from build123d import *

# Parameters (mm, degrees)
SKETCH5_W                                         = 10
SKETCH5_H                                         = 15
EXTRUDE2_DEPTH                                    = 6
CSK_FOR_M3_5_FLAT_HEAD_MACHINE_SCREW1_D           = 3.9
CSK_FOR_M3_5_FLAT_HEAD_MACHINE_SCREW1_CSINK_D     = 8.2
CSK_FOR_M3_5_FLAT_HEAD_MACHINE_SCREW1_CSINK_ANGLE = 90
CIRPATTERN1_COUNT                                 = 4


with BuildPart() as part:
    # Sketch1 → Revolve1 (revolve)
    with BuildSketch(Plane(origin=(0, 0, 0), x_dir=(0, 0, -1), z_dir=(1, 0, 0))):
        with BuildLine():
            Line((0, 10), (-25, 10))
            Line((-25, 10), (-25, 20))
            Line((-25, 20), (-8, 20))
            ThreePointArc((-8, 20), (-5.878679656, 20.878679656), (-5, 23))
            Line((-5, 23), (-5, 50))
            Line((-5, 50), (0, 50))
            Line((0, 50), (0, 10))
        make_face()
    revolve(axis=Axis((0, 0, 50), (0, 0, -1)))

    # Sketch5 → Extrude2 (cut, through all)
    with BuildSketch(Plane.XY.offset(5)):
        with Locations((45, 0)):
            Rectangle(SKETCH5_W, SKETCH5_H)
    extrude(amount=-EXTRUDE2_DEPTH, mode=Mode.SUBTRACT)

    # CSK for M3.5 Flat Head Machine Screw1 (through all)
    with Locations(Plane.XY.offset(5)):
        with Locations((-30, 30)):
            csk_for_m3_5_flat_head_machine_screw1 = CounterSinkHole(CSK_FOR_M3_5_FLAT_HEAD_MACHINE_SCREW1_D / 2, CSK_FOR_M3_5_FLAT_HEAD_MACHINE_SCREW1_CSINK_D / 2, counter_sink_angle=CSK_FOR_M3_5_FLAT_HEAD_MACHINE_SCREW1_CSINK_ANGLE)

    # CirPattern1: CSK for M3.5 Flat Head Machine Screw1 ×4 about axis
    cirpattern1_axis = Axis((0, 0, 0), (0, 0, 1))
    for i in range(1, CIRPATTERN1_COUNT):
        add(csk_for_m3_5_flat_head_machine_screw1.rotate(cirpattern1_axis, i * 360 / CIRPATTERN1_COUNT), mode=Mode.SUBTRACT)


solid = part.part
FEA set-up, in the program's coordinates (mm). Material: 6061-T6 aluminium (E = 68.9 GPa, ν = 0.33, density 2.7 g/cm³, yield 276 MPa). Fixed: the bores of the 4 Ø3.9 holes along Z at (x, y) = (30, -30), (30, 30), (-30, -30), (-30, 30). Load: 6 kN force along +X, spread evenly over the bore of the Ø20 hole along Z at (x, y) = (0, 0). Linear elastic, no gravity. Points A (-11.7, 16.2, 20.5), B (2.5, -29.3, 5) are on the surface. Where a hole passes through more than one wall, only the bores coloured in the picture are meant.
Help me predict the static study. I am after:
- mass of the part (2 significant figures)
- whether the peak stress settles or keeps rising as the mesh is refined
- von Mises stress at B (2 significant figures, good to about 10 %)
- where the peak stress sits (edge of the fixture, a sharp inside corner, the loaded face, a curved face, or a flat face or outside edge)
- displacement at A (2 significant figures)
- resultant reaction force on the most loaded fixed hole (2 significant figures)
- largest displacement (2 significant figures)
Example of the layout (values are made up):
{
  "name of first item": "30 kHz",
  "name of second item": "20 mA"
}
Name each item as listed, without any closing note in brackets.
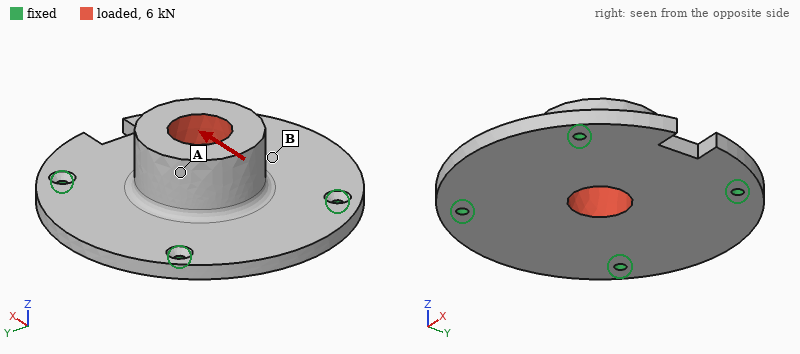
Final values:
{
  "mass of the part": "150 g",
  "whether the peak stress settles or keeps rising as the mesh is refined": "keeps rising",
  "von Mises stress at B": "24 MPa",
  "where the peak stress sits": "edge of the fixture",
  "displacement at A": "45 µm",
  "resultant reaction force on the most loaded fixed hole": "1.8 kN",
  "largest displacement": "61 µm"
}
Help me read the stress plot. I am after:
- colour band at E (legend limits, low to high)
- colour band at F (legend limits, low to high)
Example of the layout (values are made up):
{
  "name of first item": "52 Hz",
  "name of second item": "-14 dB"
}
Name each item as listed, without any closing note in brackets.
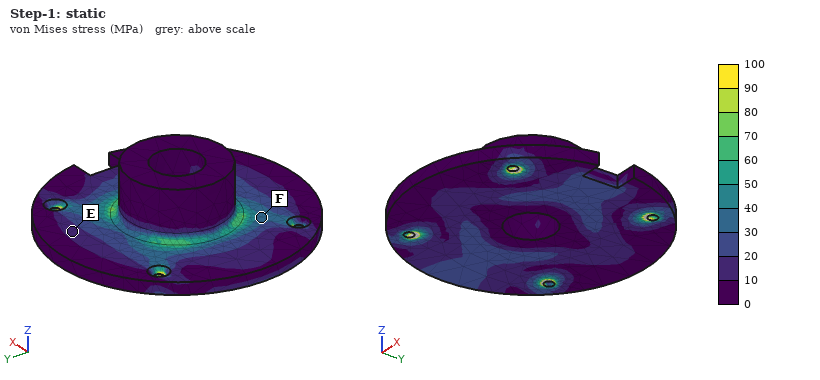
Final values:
{
  "colour band at E": "10 to 20 MPa",
  "colour band at F": "30 to 40 MPa"
}
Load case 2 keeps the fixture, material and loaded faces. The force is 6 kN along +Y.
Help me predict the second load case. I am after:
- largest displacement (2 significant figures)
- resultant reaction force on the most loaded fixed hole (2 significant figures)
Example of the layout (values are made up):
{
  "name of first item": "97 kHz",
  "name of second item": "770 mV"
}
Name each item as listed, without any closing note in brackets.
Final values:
{
  "largest displacement": "60 µm",
  "resultant reaction force on the most loaded fixed hole": "1.7 kN"
}
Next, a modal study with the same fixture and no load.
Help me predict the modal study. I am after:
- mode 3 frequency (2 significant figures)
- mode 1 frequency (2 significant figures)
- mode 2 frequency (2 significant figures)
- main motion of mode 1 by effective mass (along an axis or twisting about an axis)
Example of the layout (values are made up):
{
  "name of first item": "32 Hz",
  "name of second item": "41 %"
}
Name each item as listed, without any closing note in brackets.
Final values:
{
  "mode 3 frequency": "4800 Hz",
  "mode 1 frequency": "3700 Hz",
  "mode 2 frequency": "4700 Hz",
  "main motion of mode 1 by effective mass": "along Z"
}
